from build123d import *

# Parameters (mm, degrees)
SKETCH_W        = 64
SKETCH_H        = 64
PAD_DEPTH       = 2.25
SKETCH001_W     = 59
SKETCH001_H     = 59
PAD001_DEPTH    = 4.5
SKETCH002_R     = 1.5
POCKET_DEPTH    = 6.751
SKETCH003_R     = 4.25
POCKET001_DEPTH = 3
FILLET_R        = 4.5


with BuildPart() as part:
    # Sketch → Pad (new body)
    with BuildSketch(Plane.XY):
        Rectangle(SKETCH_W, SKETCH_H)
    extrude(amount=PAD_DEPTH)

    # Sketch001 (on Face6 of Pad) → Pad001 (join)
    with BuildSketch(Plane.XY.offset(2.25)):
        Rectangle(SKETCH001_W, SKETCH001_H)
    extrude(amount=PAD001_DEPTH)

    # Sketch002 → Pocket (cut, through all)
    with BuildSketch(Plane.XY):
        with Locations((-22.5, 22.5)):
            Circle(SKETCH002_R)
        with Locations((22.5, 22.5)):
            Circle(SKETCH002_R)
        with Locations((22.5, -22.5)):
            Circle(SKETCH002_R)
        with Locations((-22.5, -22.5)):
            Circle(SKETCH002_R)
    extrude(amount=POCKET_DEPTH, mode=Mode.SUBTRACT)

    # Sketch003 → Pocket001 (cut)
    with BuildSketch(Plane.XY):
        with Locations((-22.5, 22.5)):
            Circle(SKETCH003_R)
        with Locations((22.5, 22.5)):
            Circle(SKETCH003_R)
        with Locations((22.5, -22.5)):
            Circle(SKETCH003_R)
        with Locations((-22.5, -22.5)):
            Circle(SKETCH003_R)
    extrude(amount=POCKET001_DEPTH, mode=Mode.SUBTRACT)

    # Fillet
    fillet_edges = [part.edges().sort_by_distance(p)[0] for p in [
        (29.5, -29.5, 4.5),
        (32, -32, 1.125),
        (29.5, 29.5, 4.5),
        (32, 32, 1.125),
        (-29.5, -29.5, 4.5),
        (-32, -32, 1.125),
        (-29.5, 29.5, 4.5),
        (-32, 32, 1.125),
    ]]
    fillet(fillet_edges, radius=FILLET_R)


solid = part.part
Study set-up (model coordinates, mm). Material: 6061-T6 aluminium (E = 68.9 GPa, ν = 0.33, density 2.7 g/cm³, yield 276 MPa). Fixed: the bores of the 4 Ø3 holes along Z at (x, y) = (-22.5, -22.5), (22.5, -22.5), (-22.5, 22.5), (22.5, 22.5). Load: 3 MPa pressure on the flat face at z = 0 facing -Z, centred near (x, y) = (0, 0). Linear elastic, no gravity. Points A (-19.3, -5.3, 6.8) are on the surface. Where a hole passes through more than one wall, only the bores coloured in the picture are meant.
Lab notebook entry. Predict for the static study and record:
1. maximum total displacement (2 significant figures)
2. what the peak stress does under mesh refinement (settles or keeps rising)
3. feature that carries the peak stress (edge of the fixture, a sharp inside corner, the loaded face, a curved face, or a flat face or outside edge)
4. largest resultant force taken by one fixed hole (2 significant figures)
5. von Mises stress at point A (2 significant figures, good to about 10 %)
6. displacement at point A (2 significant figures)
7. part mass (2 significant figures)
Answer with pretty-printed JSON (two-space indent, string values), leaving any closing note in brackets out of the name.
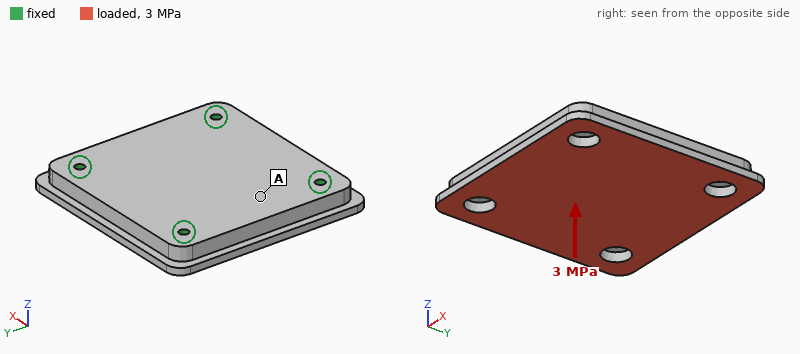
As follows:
{
  "maximum total displacement": "82 µm",
  "what the peak stress does under mesh refinement": "keeps rising",
  "feature that carries the peak stress": "edge of the fixture",
  "largest resultant force taken by one fixed hole": "3.3 kN",
  "von Mises stress at point A": "43 MPa",
  "displacement at point A": "57 µm",
  "part mass": "65 g"
}
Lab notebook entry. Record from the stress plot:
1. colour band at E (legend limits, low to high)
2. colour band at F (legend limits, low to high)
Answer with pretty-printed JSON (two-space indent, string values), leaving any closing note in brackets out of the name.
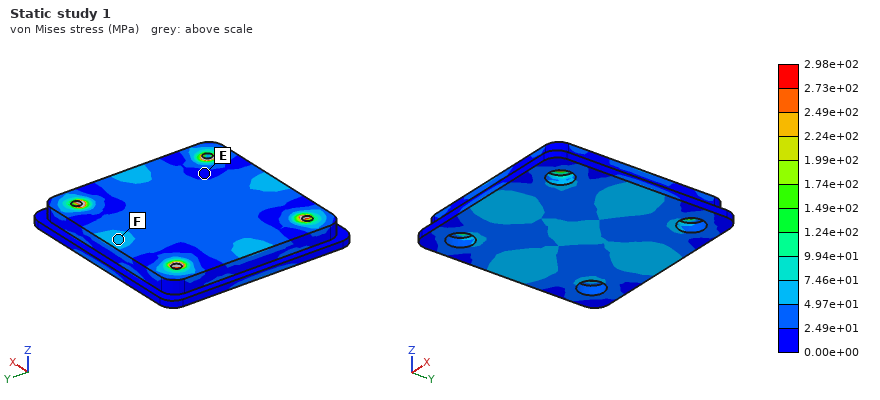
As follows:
{
  "colour band at E": "0.00e+00 to 2.49e+01 MPa",
  "colour band at F": "4.97e+01 to 7.46e+01 MPa"
}
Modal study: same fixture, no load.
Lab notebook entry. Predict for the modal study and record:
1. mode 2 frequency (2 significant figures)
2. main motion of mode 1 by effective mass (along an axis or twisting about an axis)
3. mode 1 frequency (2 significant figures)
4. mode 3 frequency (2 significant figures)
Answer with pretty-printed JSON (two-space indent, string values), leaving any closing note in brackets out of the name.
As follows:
{
  "mode 2 frequency": "12 kHz",
  "main motion of mode 1 by effective mass": "along Z",
  "mode 1 frequency": "8400 Hz",
  "mode 3 frequency": "13 kHz"
}
